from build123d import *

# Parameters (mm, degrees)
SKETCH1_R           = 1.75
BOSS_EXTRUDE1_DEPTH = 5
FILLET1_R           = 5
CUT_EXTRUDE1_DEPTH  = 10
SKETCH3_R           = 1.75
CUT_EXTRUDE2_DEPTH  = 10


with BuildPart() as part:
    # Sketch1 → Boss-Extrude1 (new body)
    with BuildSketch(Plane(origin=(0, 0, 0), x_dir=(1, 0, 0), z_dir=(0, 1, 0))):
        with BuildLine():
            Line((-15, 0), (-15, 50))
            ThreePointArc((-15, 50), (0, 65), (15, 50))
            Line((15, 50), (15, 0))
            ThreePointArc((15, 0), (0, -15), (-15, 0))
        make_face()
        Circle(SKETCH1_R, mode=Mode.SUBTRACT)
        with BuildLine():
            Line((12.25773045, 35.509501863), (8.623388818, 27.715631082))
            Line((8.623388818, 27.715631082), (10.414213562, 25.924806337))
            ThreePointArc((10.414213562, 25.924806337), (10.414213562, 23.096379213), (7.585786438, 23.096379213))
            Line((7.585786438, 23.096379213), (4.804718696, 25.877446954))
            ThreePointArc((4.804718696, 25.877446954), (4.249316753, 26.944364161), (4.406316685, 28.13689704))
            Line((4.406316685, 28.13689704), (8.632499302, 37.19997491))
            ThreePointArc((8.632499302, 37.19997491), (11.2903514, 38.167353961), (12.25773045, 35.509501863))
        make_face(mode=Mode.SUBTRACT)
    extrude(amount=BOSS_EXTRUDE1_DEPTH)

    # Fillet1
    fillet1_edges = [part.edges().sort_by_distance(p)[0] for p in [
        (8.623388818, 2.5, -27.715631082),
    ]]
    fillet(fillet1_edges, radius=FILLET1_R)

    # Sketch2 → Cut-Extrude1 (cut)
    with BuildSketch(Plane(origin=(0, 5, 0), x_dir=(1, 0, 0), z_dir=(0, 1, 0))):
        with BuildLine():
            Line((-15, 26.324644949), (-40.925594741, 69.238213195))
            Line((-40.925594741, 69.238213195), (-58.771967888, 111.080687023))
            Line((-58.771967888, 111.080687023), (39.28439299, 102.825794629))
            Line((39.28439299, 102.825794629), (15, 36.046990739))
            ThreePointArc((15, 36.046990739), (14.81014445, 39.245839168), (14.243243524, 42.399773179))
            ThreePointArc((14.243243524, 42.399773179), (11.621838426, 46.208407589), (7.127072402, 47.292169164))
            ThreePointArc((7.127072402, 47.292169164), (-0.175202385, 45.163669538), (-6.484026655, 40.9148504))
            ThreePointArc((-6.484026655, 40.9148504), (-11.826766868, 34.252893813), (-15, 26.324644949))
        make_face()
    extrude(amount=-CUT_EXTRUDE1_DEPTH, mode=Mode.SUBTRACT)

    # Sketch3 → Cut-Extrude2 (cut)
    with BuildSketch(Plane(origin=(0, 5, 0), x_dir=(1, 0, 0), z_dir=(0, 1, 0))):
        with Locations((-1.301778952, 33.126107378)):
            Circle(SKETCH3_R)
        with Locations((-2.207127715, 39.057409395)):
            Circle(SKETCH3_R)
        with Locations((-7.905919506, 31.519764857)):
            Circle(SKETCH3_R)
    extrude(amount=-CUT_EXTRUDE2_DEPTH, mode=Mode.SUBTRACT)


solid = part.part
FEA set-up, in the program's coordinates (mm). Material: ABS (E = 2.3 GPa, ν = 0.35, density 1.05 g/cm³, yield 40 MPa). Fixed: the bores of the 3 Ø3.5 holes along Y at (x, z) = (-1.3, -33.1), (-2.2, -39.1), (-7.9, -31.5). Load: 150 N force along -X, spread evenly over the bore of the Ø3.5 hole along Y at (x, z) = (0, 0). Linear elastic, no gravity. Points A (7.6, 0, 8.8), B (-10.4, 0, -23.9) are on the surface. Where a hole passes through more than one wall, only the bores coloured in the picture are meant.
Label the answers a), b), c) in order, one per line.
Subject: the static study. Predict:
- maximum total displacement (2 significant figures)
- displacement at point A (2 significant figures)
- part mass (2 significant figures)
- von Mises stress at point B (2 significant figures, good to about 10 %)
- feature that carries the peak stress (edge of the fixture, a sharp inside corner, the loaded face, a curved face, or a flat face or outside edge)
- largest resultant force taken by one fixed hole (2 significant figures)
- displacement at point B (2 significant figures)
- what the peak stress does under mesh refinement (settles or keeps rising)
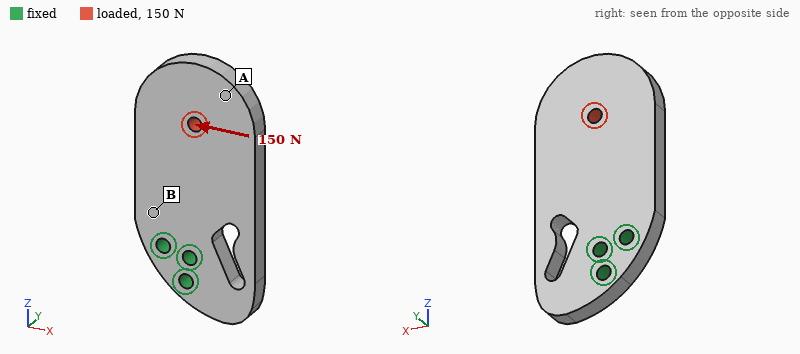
a) 0.41 mm
b) 0.37 mm
c) 8.0 g
d) 5.5 MPa
e) edge of the fixture
f) 390 N
g) 0.063 mm
h) keeps rising
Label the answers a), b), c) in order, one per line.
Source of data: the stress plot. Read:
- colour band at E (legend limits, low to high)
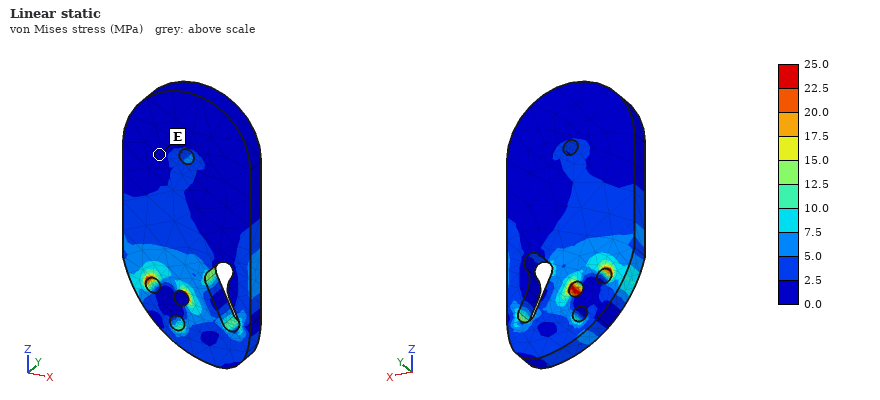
a) 0.0 to 2.5 MPa
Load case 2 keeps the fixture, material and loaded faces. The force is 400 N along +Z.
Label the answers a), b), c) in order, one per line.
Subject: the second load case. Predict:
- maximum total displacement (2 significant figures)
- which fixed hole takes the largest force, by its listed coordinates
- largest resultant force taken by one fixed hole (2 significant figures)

a) 0.15 mm
b) (-1.3, -33.1)
c) 300 N
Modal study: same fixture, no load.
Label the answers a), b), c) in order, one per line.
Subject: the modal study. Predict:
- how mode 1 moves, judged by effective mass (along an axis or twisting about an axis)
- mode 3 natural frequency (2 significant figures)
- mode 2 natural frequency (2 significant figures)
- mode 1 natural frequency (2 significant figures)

a) along Y
b) 1700 Hz
c) 1600 Hz
d) 550 Hz
